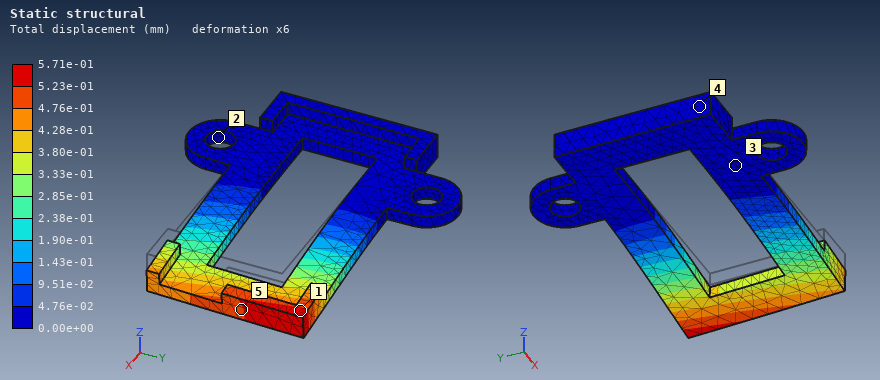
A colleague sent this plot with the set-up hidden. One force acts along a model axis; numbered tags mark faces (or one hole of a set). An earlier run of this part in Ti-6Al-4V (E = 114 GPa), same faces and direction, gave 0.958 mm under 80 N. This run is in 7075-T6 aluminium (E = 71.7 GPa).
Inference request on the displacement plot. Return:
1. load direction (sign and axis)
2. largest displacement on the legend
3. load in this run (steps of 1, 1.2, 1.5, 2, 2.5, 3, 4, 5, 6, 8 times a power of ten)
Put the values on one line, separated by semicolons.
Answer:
-Z; 5.71e-01 mm; 30 N
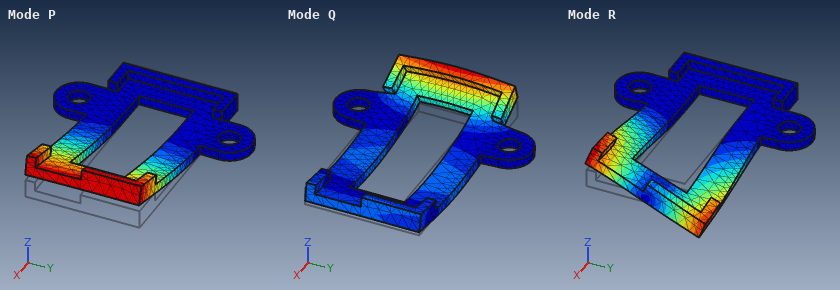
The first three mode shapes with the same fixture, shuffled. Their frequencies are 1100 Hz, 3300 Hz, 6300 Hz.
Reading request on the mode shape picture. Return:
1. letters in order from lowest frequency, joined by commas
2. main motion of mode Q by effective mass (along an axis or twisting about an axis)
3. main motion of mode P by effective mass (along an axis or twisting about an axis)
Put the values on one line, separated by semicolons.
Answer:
P, R, Q; along Z; along Z
